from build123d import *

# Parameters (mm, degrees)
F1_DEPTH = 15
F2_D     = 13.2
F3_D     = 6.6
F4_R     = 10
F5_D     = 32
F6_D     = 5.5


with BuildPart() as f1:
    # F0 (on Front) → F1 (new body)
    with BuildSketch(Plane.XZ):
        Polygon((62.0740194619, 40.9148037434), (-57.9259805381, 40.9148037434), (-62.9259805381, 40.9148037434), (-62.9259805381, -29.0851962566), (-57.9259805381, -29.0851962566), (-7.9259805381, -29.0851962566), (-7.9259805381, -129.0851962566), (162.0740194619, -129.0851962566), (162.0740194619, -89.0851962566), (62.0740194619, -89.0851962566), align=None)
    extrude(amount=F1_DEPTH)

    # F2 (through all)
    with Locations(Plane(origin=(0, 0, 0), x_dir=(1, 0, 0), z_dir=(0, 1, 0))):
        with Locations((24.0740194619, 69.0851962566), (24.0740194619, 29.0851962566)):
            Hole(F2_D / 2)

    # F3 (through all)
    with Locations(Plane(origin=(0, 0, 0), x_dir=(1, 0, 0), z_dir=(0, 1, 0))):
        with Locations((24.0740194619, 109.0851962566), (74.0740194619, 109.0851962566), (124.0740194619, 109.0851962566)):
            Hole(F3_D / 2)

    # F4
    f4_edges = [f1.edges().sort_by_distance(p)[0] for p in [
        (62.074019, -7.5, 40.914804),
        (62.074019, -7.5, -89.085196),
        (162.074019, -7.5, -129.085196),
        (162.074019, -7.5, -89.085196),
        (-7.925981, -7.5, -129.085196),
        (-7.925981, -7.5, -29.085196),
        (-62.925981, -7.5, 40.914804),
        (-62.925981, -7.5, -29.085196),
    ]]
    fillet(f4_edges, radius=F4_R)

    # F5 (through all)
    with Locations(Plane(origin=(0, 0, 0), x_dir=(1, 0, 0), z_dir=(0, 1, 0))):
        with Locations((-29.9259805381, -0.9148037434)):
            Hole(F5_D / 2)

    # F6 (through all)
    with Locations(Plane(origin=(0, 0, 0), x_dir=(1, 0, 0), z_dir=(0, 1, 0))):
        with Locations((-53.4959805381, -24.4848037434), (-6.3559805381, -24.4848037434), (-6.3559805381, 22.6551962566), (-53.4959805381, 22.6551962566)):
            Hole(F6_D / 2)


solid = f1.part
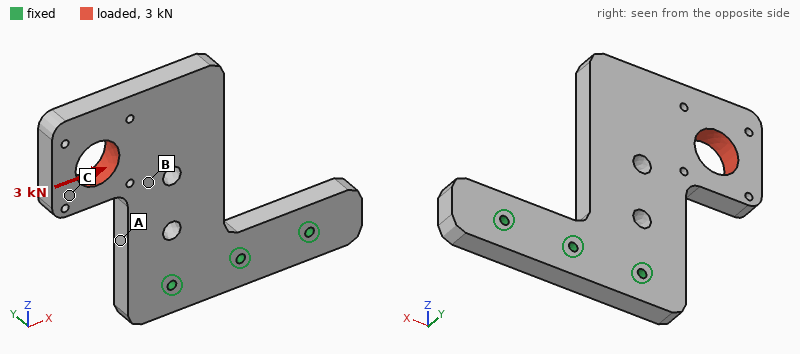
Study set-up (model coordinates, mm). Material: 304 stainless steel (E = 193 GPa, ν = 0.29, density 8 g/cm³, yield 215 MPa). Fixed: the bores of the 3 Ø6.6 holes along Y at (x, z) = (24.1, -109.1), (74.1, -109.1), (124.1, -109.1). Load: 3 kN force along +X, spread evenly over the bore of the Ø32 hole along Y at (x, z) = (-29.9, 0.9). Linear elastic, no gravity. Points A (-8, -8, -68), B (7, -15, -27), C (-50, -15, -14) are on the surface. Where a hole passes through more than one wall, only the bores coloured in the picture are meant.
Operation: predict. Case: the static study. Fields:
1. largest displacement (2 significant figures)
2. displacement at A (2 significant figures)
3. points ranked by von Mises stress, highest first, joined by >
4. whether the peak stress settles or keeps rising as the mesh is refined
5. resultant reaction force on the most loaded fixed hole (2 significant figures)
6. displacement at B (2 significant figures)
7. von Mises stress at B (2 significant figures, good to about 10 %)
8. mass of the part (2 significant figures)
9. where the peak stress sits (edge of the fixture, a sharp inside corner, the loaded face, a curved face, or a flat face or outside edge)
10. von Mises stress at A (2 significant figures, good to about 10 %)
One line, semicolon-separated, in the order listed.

51 µm; 13 µm; A > B > C; keeps rising; 6.2 kN; 22 µm; 8.5 MPa; 2.2 kg; edge of the fixture; 15 MPa
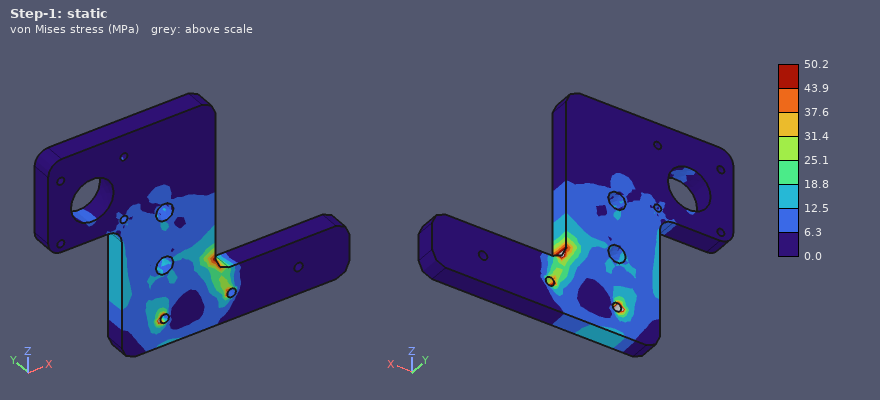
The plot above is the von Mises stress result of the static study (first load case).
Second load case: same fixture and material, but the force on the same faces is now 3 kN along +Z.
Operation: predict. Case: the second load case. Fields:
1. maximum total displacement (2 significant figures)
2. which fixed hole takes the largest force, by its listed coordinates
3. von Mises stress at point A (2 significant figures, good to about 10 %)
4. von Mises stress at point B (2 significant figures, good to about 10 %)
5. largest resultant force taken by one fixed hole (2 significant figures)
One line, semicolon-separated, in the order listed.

44 µm; (24.1, -109.1); 15 MPa; 7.9 MPa; 5.9 kN
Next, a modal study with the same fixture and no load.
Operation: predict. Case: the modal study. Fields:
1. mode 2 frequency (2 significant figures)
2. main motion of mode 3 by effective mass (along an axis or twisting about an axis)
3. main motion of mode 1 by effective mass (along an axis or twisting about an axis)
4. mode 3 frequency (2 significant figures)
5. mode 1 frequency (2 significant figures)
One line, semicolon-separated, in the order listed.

1000 Hz; along X; along Y; 1300 Hz; 380 Hz
